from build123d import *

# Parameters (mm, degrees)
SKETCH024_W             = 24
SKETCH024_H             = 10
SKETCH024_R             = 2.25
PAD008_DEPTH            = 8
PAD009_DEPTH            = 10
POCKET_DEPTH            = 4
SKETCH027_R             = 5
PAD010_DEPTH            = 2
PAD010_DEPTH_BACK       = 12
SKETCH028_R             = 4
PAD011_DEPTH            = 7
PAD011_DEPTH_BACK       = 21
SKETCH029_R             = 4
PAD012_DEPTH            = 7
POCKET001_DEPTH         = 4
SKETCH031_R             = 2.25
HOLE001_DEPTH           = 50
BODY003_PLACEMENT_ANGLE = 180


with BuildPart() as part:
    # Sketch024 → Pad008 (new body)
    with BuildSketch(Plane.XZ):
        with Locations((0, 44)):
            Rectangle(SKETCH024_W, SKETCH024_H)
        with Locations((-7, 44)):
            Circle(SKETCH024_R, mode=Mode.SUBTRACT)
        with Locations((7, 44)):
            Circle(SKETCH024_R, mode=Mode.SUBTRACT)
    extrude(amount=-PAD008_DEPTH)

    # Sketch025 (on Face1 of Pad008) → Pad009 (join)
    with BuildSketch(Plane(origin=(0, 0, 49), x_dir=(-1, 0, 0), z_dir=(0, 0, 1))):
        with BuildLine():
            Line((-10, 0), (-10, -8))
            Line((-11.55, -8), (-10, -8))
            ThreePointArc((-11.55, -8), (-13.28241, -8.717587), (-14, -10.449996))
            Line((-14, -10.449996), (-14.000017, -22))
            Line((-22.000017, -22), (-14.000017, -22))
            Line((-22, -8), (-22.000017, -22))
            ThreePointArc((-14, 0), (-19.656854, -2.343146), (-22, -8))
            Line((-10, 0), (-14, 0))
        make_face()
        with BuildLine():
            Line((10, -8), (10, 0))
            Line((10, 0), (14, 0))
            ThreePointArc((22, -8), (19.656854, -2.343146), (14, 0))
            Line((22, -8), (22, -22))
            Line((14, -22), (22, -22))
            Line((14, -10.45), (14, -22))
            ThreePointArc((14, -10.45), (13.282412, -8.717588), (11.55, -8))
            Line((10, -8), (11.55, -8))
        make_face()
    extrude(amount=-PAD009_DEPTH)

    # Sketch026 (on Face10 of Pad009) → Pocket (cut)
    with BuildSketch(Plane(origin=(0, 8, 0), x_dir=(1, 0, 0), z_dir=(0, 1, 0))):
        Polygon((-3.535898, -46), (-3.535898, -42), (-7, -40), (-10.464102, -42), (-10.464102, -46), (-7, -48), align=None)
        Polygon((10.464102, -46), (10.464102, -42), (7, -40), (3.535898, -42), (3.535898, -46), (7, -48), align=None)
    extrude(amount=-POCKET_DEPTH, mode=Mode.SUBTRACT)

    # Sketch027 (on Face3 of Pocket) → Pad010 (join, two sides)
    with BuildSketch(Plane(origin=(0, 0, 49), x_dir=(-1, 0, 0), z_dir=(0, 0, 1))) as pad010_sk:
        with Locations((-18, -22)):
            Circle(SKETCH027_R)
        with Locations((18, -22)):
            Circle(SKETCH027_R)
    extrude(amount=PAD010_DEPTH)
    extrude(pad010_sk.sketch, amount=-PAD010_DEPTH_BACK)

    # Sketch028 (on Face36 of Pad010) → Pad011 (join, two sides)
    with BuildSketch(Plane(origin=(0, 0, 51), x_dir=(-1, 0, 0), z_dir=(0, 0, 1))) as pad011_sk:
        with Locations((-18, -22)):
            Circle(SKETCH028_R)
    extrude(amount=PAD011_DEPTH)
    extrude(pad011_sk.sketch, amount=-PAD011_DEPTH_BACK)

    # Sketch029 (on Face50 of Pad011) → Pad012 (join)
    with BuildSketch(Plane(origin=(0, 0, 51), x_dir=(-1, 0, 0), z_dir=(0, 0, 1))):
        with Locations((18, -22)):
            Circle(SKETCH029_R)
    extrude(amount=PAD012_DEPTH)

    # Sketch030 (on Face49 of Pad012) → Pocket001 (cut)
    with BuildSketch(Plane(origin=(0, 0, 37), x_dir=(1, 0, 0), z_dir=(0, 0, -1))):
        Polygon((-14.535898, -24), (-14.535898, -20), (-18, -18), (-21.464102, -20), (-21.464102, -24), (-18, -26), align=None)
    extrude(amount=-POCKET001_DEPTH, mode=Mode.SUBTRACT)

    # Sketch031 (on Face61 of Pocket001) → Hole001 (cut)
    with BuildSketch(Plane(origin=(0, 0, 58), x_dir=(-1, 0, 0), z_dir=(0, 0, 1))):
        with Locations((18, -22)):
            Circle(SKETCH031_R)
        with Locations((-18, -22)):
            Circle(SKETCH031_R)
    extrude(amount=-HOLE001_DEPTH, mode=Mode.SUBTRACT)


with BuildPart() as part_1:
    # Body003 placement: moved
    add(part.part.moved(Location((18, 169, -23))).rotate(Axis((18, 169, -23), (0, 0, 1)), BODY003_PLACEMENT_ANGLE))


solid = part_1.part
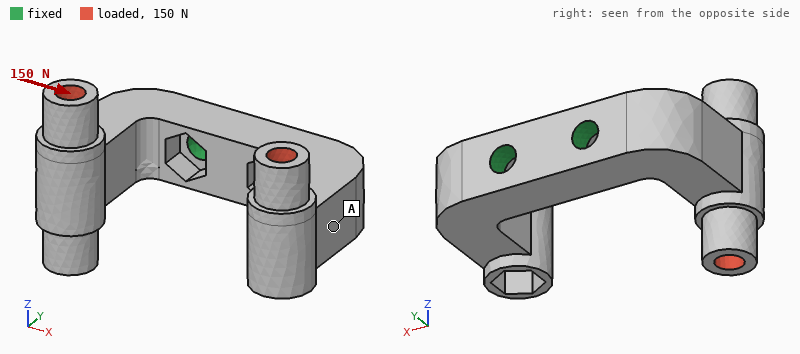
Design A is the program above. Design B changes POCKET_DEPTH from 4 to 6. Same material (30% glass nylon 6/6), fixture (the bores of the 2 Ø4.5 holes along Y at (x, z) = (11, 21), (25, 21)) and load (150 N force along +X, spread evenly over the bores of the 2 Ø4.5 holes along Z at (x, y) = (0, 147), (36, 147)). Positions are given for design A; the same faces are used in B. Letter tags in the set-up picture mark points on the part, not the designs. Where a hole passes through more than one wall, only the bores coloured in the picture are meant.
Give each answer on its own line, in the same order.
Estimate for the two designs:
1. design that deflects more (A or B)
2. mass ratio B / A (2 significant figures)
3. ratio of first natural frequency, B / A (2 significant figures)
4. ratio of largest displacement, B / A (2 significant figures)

B
0.98
0.77
1.3
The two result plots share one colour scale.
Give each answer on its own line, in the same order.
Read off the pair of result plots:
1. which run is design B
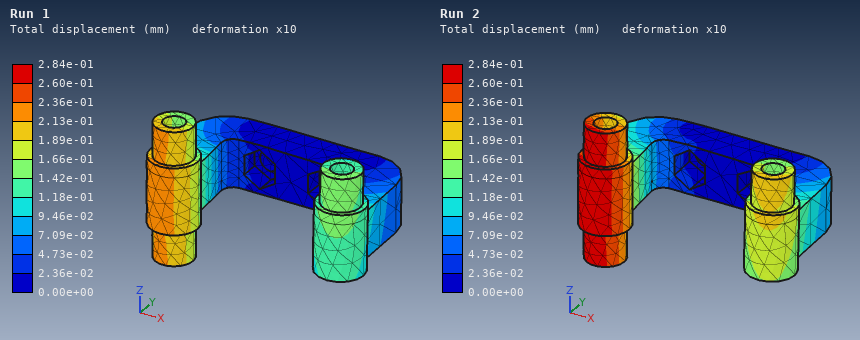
Run 2
